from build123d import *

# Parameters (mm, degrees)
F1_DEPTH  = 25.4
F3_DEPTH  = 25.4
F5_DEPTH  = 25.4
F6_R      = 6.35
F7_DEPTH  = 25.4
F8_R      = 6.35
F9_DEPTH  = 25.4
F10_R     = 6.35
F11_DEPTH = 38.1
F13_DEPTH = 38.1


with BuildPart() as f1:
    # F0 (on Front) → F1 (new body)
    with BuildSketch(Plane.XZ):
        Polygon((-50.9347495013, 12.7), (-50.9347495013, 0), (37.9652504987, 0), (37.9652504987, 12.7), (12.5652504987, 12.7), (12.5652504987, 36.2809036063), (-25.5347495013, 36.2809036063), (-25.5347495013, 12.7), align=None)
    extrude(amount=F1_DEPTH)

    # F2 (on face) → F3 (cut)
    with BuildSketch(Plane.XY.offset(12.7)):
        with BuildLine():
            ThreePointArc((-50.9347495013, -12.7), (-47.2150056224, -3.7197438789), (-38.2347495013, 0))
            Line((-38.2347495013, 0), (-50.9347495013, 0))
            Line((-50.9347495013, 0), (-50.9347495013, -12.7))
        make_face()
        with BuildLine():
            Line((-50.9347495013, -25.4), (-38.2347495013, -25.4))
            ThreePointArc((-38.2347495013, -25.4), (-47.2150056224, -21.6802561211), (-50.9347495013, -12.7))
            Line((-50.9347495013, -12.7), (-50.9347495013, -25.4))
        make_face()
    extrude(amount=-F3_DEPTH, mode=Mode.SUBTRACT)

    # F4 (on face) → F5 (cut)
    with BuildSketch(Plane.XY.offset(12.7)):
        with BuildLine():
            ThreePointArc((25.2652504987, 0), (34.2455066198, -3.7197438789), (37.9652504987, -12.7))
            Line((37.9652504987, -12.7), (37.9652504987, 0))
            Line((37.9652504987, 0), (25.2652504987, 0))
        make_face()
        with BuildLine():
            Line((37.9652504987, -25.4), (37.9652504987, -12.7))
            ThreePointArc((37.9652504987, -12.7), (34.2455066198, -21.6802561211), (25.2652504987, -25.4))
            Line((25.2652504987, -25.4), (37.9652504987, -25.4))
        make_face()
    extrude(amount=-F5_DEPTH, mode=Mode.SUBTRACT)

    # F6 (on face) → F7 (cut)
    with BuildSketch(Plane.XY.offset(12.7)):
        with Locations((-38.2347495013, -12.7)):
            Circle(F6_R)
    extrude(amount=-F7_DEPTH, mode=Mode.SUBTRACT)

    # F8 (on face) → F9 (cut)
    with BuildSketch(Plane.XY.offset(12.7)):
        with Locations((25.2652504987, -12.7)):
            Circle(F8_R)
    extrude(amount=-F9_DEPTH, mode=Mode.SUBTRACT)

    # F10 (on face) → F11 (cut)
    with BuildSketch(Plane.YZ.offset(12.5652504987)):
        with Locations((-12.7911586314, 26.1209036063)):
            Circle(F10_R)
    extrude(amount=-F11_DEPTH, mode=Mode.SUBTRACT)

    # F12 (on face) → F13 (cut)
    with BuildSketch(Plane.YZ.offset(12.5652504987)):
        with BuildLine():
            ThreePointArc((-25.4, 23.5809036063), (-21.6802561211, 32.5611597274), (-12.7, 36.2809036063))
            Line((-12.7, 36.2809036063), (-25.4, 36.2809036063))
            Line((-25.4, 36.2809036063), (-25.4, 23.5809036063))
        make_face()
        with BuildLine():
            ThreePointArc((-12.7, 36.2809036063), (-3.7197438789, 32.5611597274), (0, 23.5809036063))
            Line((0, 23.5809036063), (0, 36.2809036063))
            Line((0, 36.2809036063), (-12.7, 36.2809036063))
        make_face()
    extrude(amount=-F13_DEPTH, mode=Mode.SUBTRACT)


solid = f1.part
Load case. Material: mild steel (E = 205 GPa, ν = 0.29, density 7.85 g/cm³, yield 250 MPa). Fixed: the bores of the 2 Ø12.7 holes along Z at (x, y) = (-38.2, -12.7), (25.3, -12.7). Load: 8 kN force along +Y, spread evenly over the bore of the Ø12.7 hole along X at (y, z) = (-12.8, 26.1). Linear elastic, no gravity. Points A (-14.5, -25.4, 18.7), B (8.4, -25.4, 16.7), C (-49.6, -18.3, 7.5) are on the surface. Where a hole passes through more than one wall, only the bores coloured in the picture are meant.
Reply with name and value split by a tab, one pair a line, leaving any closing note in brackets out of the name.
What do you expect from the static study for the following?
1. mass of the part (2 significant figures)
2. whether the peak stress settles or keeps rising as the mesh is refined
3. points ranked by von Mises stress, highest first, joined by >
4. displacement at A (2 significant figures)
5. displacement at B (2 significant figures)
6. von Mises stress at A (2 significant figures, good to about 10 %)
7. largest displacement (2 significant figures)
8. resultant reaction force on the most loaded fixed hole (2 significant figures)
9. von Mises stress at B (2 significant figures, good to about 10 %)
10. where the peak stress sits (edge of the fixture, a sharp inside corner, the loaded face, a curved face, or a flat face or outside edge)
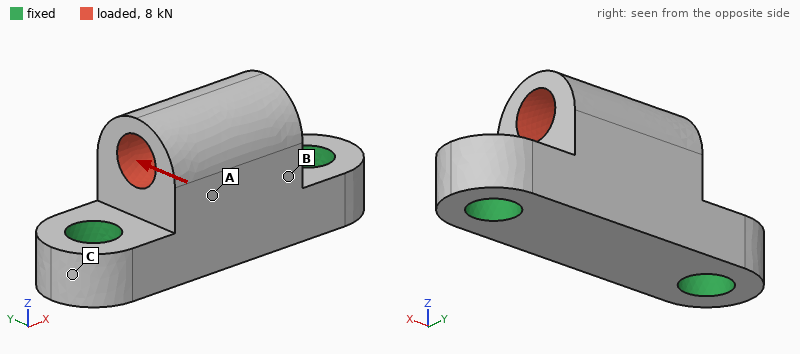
mass of the part	310 g
whether the peak stress settles or keeps rising as the mesh is refined	keeps rising
points ranked by von Mises stress, highest first, joined by >	B > A > C
displacement at A	20 µm
displacement at B	18 µm
von Mises stress at A	30 MPa
largest displacement	37 µm
resultant reaction force on the most loaded fixed hole	4.0 kN
von Mises stress at B	45 MPa
where the peak stress sits	edge of the fixture
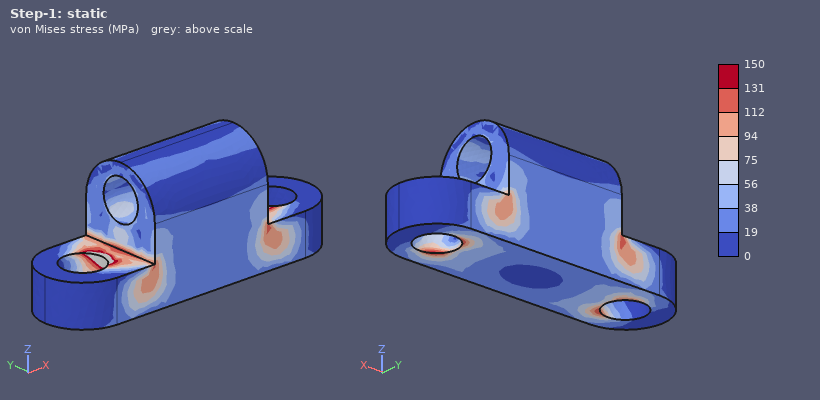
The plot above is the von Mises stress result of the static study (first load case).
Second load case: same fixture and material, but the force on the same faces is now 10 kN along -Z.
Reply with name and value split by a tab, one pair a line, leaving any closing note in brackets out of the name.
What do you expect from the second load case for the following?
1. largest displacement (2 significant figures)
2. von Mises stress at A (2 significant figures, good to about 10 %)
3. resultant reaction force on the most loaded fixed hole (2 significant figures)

largest displacement	7.6 µm
von Mises stress at A	12 MPa
resultant reaction force on the most loaded fixed hole	5.3 kN
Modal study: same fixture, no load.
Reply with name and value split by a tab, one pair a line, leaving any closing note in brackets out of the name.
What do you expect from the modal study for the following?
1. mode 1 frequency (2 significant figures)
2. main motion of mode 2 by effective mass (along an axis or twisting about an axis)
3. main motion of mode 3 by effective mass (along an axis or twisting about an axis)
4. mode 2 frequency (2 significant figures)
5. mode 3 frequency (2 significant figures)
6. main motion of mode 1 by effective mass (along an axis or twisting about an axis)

mode 1 frequency	8300 Hz
main motion of mode 2 by effective mass	along Z
main motion of mode 3 by effective mass	along X
mode 2 frequency	15 kHz
mode 3 frequency	18 kHz
main motion of mode 1 by effective mass	along Y
